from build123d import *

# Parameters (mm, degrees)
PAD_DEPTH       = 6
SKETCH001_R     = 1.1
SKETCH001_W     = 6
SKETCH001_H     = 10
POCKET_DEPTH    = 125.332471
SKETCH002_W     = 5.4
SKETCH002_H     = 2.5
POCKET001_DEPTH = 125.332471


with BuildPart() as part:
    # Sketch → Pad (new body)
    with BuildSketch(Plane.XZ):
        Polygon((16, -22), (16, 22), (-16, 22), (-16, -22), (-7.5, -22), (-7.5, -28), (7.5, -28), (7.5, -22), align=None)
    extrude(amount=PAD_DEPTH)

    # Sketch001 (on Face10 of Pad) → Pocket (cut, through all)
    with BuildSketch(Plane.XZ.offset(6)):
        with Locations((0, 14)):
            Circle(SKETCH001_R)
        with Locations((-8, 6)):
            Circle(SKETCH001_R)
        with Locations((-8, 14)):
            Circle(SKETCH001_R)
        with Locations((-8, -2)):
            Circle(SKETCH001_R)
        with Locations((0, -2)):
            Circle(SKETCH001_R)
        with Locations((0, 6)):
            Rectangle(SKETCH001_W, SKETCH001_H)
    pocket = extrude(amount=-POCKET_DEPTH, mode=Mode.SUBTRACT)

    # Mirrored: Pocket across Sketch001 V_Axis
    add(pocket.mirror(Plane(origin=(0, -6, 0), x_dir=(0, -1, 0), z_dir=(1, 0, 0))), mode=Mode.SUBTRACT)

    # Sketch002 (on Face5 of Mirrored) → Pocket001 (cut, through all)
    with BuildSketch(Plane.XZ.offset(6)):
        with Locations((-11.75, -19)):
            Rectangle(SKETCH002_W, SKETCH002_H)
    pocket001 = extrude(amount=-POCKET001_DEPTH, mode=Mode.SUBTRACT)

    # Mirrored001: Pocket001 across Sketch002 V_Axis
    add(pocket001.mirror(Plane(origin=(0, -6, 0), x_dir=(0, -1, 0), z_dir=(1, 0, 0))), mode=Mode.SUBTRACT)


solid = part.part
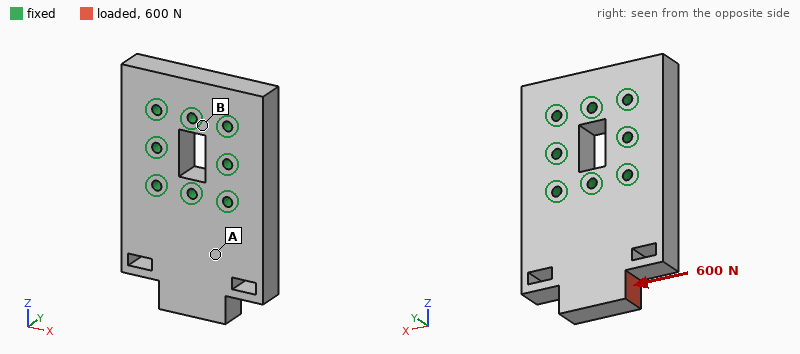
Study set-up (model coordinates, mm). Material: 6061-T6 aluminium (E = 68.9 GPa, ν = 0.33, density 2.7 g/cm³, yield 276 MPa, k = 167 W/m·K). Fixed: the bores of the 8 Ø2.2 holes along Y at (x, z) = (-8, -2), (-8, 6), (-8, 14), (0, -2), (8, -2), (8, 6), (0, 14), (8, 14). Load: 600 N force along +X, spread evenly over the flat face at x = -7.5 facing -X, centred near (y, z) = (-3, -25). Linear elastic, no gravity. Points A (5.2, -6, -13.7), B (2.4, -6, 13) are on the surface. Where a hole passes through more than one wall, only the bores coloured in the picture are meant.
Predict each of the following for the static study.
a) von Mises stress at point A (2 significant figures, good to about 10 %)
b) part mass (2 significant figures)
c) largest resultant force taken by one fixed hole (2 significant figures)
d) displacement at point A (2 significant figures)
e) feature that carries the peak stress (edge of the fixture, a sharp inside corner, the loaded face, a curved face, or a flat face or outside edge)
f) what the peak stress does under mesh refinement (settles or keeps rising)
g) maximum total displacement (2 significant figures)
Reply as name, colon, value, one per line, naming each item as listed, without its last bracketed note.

von Mises stress at point A: 8.2 MPa
part mass: 22 g
largest resultant force taken by one fixed hole: 540 N
displacement at point A: 3.1 µm
feature that carries the peak stress: edge of the fixture
what the peak stress does under mesh refinement: keeps rising
maximum total displacement: 11 µm
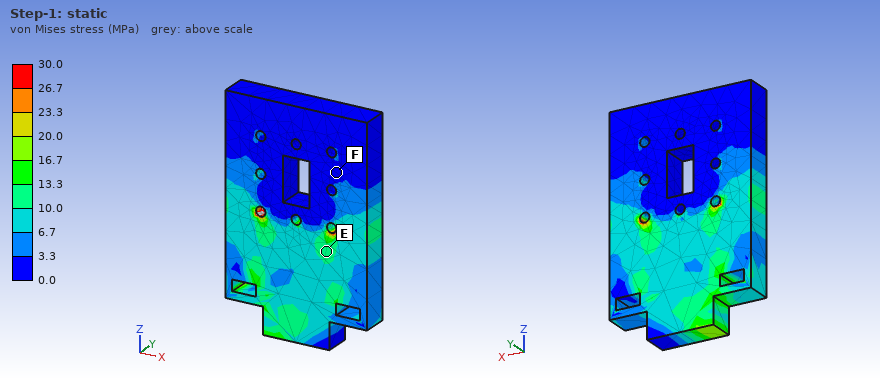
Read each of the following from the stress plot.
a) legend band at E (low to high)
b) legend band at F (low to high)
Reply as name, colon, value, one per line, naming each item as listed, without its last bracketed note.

legend band at E: 10.0 to 13.3 MPa
legend band at F: 0.0 to 3.3 MPa
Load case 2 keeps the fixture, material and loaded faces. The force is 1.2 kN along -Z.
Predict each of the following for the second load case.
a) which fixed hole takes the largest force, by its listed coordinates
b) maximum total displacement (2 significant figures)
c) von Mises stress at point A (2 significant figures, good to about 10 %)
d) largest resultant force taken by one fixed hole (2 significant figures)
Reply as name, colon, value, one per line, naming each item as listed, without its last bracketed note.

which fixed hole takes the largest force, by its listed coordinates: (-8, -2)
maximum total displacement: 17 µm
von Mises stress at point A: 3.4 MPa
largest resultant force taken by one fixed hole: 690 N
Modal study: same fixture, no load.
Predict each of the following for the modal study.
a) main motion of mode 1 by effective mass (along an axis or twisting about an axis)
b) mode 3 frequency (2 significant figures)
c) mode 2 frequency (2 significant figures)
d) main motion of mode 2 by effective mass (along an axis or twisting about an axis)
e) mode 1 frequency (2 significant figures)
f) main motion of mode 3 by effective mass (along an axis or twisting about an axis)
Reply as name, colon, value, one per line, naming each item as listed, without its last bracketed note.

main motion of mode 1 by effective mass: along Y
mode 3 frequency: 23 kHz
mode 2 frequency: 17 kHz
main motion of mode 2 by effective mass: twisting about Z
mode 1 frequency: 8500 Hz
main motion of mode 3 by effective mass: along X
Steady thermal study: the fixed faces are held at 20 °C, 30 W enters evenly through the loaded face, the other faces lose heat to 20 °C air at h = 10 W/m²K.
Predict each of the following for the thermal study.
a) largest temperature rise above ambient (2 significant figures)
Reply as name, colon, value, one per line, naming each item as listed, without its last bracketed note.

largest temperature rise above ambient: 49 K
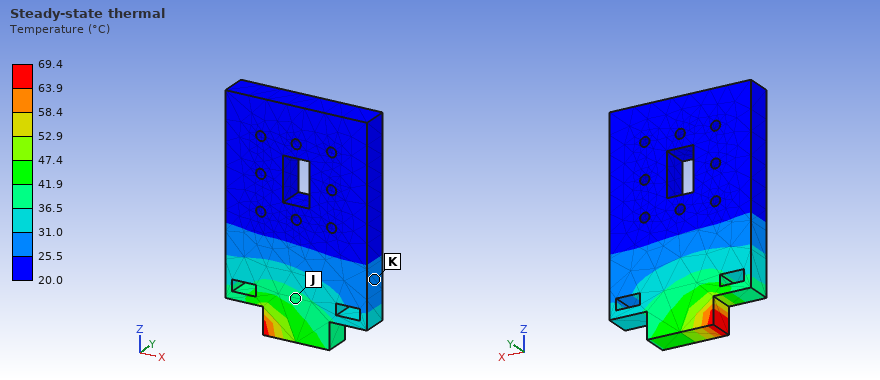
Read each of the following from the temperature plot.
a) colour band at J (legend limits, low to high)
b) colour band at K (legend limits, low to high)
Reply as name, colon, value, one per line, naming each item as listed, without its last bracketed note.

colour band at J: 36.5 to 41.9 °C
colour band at K: 25.5 to 31.0 °C
